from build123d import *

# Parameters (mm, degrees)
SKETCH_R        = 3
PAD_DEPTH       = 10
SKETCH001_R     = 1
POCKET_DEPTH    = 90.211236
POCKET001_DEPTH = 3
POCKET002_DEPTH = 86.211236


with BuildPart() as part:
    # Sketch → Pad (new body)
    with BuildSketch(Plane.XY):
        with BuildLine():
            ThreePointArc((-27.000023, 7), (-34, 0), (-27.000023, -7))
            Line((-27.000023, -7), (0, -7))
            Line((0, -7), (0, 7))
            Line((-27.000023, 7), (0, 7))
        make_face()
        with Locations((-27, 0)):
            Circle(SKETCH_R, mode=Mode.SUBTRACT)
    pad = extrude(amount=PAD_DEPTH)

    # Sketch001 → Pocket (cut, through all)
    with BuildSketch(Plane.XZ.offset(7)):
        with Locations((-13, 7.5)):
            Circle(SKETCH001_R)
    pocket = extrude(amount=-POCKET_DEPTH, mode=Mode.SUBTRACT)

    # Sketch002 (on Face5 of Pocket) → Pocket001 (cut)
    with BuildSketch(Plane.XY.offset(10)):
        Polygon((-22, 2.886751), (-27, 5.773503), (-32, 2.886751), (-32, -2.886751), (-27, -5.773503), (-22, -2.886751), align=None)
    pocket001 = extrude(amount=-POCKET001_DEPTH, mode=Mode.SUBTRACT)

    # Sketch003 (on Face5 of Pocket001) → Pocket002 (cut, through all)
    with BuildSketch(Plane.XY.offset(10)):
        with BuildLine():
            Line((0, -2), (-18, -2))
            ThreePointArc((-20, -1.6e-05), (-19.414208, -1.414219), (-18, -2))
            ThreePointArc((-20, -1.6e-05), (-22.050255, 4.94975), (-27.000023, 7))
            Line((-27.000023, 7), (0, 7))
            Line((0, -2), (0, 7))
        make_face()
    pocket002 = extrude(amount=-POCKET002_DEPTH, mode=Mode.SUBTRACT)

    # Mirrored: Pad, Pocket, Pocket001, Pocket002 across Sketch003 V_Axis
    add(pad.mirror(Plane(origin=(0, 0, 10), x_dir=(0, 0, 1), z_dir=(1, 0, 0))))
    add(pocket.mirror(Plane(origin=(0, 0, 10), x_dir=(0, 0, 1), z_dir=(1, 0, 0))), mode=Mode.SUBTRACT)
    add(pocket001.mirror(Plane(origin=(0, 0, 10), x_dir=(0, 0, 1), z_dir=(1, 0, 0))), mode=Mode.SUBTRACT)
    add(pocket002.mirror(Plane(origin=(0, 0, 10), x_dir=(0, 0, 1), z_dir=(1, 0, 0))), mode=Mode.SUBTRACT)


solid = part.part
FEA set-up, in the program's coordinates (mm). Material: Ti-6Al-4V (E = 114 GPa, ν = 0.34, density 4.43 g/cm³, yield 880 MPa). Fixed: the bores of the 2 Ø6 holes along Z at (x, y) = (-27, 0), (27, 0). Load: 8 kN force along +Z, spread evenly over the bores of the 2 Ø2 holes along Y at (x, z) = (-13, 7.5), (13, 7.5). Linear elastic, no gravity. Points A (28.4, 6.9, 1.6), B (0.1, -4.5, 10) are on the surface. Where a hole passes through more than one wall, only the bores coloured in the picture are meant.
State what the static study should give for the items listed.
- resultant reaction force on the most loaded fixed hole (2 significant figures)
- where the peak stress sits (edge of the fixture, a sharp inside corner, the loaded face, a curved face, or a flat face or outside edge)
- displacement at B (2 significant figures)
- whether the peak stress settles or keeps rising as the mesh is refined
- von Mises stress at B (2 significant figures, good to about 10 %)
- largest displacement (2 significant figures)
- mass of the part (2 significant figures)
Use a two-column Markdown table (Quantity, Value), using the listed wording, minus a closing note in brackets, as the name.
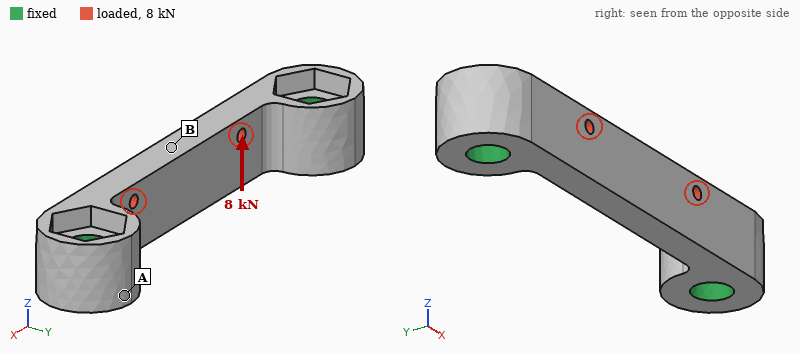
| Quantity | Value |
|---|---|
| resultant reaction force on the most loaded fixed hole | 4.1 kN |
| where the peak stress sits | edge of the fixture |
| displacement at B | 0.098 mm |
| whether the peak stress settles or keeps rising as the mesh is refined | keeps rising |
| von Mises stress at B | 190 MPa |
| largest displacement | 0.10 mm |
| mass of the part | 19 g |
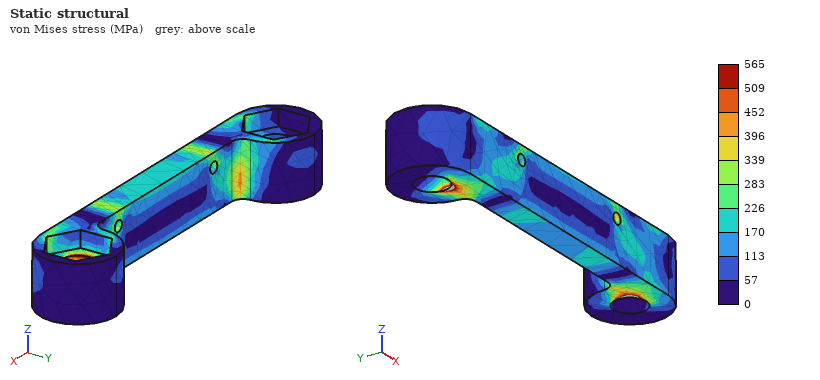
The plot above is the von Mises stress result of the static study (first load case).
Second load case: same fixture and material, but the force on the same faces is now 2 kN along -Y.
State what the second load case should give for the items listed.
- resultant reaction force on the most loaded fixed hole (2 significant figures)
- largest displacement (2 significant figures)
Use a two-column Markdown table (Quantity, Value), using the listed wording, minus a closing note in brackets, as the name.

| Quantity | Value |
|---|---|
| resultant reaction force on the most loaded fixed hole | 1.1 kN |
| largest displacement | 46 µm |
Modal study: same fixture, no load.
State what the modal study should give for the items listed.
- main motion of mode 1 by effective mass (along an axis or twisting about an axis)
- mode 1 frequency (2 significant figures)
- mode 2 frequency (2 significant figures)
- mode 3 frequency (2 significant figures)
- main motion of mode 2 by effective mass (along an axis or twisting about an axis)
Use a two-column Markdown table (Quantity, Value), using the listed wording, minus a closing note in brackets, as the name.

| Quantity | Value |
|---|---|
| main motion of mode 1 by effective mass | along Y |
| mode 1 frequency | 12 kHz |
| mode 2 frequency | 15 kHz |
| mode 3 frequency | 26 kHz |
| main motion of mode 2 by effective mass | along Z |
